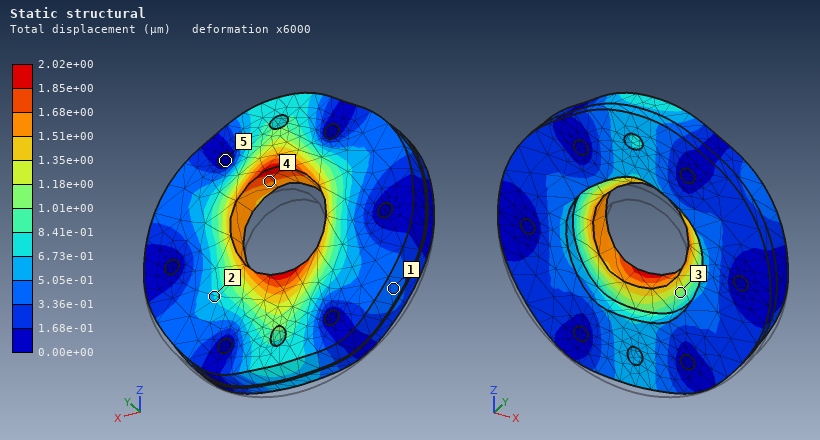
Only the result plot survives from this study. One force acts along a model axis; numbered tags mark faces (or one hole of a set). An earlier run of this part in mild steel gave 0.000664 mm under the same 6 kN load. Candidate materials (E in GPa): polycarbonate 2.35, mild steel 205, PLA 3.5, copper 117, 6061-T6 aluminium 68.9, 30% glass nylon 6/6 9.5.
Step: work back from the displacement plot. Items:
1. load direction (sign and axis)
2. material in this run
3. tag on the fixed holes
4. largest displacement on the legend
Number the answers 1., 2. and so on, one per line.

1. +Z
2. 6061-T6 aluminium
3. 5
4. 2.02e+00 µm
